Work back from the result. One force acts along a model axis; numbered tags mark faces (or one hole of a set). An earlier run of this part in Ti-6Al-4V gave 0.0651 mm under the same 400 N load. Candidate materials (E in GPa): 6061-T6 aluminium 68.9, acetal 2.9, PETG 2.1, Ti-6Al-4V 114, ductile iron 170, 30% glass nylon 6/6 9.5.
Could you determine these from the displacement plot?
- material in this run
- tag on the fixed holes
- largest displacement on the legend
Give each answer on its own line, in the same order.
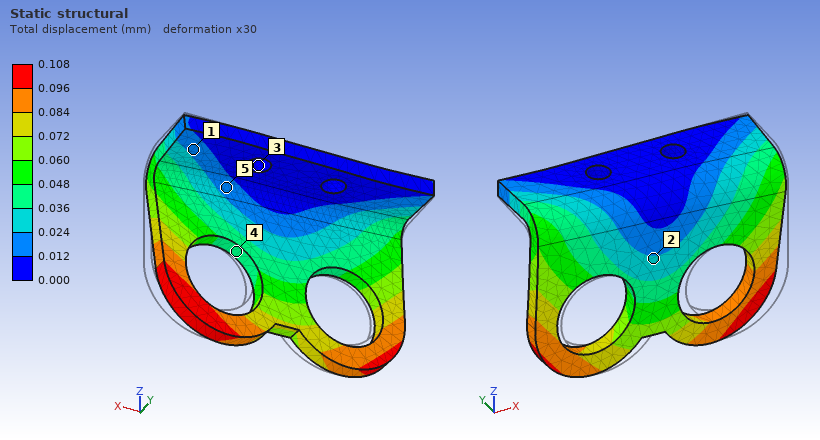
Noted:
6061-T6 aluminium
3
0.108 mm
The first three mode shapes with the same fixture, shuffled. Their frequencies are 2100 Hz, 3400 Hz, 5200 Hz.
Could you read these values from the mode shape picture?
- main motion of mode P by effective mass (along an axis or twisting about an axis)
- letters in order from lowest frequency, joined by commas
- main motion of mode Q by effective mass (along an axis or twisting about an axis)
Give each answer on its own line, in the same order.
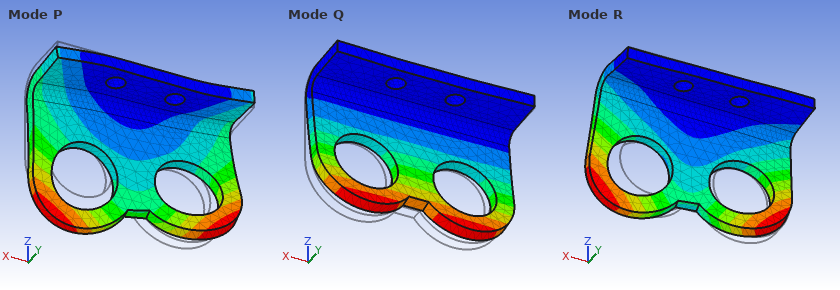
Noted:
along X
Q, R, P
along Y
